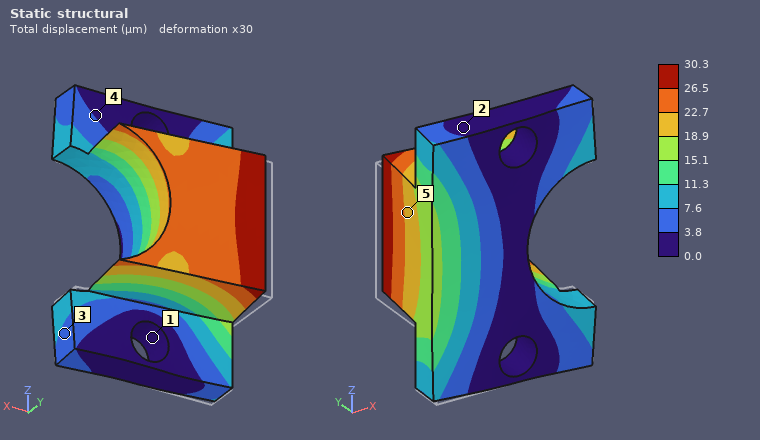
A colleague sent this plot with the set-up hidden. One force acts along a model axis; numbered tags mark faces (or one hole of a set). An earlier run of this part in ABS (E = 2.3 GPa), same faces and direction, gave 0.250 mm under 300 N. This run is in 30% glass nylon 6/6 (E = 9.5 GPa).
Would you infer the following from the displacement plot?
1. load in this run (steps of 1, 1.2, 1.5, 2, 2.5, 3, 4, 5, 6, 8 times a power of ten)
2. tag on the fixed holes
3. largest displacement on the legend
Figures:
150 N
1
30.3 µm
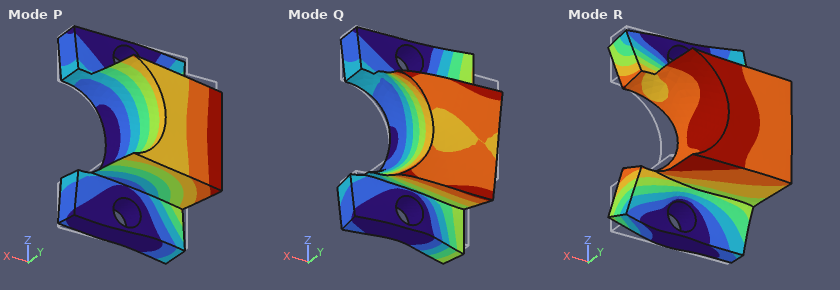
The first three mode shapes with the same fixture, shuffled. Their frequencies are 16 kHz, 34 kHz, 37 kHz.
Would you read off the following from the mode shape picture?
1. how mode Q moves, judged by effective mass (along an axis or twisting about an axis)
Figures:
along Z
